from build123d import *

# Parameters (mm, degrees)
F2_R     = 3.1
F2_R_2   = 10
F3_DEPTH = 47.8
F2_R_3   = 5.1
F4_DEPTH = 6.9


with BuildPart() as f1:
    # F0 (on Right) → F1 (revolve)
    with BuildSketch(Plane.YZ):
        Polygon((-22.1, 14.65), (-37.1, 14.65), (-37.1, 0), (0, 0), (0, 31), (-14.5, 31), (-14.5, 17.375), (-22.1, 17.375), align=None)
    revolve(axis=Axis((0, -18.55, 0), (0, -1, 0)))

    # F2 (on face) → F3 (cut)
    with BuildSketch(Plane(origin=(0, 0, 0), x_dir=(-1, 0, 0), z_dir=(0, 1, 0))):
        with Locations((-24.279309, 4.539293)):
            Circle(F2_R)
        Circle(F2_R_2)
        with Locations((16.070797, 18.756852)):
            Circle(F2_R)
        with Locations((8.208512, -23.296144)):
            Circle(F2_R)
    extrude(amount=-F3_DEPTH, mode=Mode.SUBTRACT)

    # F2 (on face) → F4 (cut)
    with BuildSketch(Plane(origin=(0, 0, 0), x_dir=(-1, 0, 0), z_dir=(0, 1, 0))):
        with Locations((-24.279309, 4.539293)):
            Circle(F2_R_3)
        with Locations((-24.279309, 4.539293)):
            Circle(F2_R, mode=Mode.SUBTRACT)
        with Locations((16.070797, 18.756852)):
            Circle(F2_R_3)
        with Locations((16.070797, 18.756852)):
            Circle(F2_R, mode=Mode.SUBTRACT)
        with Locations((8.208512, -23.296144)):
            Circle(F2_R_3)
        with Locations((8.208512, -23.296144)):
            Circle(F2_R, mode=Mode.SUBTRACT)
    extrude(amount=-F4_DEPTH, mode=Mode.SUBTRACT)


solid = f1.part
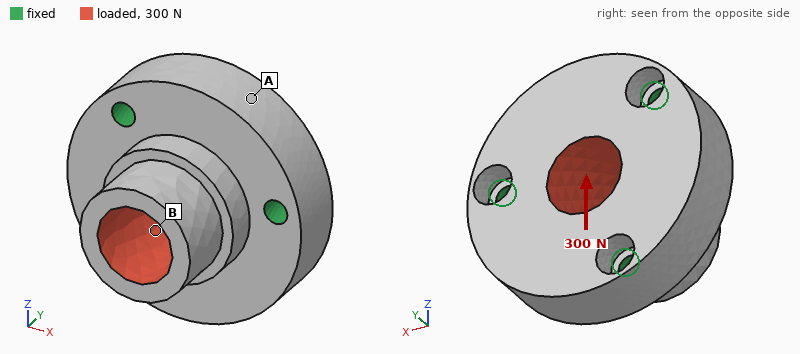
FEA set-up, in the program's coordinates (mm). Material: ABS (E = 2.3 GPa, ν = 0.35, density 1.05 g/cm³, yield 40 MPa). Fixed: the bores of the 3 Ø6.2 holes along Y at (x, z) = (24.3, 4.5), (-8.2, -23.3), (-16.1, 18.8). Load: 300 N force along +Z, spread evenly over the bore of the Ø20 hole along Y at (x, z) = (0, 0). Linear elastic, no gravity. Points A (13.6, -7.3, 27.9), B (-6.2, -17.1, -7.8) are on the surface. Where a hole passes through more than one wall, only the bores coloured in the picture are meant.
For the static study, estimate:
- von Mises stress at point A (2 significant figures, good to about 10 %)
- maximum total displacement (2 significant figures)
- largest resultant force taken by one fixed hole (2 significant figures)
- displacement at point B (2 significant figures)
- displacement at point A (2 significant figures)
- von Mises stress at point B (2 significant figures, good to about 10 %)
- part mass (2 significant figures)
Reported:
0.28 MPa
26 µm
110 N
5.8 µm
7.9 µm
0.60 MPa
49 g
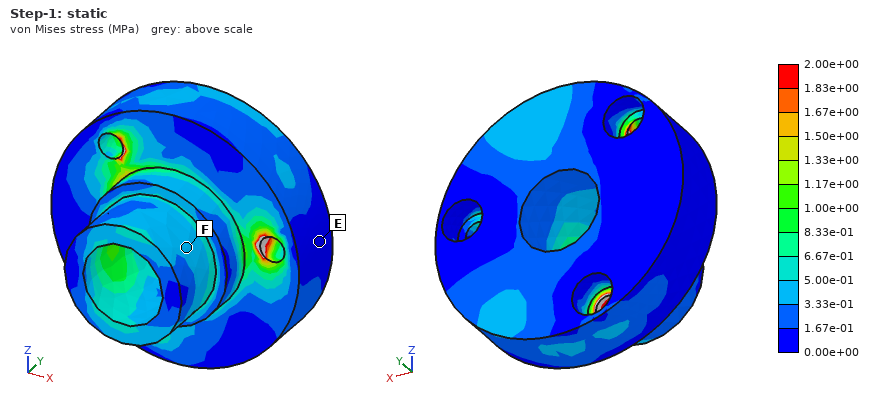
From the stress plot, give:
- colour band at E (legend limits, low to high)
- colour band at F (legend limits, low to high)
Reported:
0.00e+00 to 1.67e-01 MPa
3.33e-01 to 5.00e-01 MPa
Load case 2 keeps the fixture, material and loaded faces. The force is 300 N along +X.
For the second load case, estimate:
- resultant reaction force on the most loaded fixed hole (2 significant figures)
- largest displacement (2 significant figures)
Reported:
110 N
26 µm
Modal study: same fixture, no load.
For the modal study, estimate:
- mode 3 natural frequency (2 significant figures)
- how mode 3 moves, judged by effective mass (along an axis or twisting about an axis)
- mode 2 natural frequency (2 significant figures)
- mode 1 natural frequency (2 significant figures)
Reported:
4900 Hz
along Y
4000 Hz
3900 Hz
